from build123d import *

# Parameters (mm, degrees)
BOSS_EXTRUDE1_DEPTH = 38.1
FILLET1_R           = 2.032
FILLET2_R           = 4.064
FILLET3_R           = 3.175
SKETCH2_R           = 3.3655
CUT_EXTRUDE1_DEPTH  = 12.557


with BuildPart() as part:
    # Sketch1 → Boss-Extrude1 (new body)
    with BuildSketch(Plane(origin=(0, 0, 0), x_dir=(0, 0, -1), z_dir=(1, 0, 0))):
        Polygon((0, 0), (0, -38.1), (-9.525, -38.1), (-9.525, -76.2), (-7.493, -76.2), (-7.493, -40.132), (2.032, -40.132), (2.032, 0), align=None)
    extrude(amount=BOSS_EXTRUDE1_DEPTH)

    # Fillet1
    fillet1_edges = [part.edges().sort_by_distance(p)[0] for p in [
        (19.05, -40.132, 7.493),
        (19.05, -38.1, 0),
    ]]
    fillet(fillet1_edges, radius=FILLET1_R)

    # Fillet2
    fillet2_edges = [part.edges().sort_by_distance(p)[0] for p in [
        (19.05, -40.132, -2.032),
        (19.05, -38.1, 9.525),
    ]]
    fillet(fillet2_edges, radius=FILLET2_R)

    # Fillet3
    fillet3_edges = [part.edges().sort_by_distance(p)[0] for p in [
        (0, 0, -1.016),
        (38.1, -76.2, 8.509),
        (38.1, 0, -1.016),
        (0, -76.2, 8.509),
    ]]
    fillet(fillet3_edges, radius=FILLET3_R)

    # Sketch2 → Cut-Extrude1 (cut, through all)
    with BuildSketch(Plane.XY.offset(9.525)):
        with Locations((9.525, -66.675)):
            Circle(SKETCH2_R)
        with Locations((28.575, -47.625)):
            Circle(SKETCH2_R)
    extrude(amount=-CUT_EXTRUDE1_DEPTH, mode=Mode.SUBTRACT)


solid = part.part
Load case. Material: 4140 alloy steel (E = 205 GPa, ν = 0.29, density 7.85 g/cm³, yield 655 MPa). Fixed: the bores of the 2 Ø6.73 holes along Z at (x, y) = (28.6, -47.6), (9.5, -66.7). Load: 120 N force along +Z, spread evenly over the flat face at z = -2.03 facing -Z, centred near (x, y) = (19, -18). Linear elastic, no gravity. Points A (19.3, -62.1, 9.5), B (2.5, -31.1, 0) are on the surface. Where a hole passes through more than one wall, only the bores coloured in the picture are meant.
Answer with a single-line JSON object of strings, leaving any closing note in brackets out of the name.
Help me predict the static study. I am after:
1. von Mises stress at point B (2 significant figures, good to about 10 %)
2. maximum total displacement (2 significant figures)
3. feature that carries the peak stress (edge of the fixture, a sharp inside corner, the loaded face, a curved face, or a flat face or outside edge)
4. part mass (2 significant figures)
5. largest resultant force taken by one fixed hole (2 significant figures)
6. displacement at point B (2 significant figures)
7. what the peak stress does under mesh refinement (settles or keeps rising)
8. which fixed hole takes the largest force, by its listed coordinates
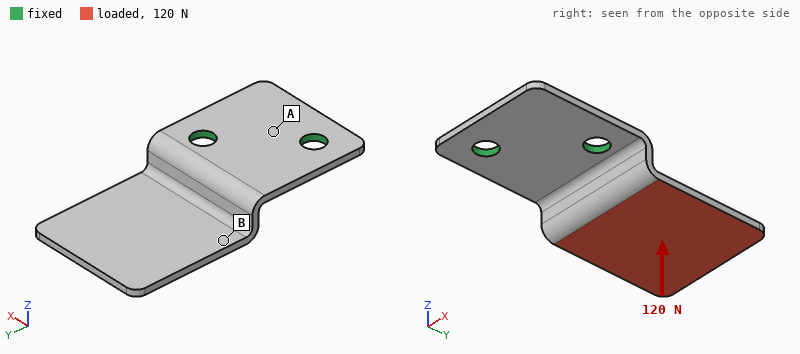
{"von Mises stress at point B": "52 MPa", "maximum total displacement": "0.52 mm", "feature that carries the peak stress": "edge of the fixture", "part mass": "49 g", "largest resultant force taken by one fixed hole": "170 N", "displacement at point B": "0.14 mm", "what the peak stress does under mesh refinement": "keeps rising", "which fixed hole takes the largest force, by its listed coordinates": "(28.6, -47.6)"}
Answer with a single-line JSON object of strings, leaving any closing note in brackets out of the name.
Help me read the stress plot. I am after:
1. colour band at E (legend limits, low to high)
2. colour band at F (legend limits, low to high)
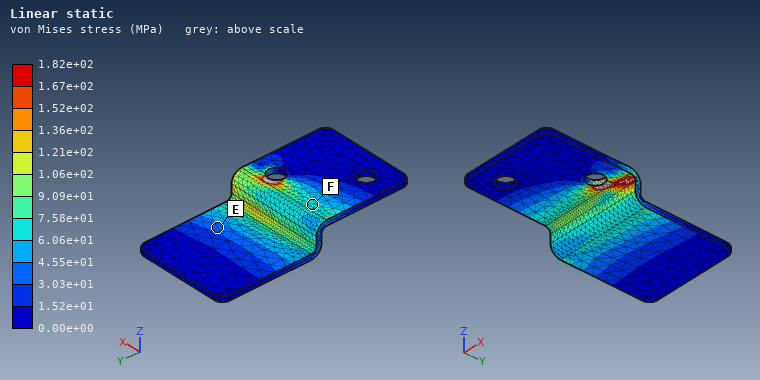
{"colour band at E": "3.03e+01 to 4.55e+01 MPa", "colour band at F": "6.06e+01 to 7.58e+01 MPa"}
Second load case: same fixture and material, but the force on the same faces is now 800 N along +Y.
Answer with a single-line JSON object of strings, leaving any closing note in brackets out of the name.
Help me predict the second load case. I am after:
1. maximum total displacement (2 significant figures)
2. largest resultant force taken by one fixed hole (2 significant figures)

{"maximum total displacement": "0.91 mm", "largest resultant force taken by one fixed hole": "450 N"}
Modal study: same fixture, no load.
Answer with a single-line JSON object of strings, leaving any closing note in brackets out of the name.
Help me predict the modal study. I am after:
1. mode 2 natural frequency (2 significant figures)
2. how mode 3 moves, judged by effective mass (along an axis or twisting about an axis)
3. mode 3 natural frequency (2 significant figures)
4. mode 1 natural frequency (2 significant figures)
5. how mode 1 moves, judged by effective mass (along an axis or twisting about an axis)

{"mode 2 natural frequency": "1800 Hz", "how mode 3 moves, judged by effective mass": "along X", "mode 3 natural frequency": "2500 Hz", "mode 1 natural frequency": "640 Hz", "how mode 1 moves, judged by effective mass": "along Z"}
